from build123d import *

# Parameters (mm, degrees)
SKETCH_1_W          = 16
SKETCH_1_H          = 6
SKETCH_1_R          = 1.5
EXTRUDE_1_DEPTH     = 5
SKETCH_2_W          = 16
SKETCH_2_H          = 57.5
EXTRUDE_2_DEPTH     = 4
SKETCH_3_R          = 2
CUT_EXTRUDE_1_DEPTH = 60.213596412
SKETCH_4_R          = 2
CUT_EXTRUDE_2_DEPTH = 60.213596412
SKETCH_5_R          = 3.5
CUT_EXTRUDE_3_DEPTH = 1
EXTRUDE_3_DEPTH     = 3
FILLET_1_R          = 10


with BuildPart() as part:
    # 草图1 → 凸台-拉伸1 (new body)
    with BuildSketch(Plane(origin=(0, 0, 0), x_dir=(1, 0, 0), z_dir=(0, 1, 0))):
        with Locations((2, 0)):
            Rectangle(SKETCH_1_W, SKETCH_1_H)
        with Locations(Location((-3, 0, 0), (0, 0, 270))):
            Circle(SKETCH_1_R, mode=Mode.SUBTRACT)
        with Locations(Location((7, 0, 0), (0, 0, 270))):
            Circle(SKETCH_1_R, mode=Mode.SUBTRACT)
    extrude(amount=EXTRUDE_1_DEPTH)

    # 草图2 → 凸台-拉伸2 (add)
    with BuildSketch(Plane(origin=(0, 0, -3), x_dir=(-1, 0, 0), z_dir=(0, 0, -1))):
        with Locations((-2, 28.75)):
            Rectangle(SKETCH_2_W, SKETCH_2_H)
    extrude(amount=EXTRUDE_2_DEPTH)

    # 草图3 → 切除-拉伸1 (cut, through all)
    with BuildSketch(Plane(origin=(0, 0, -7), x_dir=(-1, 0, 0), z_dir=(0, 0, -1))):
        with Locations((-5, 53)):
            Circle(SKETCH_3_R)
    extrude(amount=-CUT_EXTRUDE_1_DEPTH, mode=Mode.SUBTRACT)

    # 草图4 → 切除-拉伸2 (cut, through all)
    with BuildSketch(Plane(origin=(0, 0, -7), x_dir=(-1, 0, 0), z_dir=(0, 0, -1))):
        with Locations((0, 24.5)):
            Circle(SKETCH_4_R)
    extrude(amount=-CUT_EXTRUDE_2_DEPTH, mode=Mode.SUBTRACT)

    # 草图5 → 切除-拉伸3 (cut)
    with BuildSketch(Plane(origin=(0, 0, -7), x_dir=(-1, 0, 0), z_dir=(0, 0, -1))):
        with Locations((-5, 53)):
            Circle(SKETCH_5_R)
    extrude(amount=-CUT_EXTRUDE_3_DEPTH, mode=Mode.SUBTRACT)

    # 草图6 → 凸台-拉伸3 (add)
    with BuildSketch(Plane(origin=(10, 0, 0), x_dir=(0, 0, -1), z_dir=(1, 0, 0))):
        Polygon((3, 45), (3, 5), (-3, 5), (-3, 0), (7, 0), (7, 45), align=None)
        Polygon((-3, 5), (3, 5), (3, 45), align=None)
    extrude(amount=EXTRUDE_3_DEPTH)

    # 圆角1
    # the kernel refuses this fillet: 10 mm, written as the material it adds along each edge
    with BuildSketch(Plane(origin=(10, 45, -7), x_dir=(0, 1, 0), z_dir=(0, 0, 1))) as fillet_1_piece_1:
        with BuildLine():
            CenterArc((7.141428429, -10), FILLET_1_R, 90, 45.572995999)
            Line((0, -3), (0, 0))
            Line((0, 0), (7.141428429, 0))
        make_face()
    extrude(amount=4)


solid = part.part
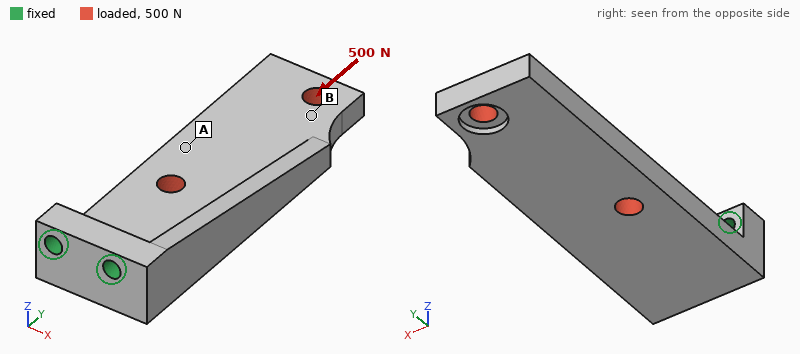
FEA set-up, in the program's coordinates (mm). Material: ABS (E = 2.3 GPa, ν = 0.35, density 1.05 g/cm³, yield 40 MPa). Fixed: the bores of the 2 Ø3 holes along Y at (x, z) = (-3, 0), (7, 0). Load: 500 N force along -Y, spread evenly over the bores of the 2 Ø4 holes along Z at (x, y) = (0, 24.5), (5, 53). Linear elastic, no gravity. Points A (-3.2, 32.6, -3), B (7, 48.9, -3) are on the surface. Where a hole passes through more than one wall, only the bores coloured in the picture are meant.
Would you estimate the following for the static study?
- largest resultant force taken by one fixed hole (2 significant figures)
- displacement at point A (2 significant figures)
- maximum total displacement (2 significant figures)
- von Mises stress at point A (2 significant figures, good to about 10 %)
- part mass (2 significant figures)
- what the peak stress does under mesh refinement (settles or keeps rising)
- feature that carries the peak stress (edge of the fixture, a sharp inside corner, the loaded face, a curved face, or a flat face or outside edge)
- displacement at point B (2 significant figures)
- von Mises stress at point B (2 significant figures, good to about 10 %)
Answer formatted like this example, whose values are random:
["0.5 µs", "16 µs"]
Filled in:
["250 N", "0.42 mm", "0.63 mm", "3.4 MPa", "5.2 g", "keeps rising", "edge of the fixture", "0.55 mm", "7.7 MPa"]
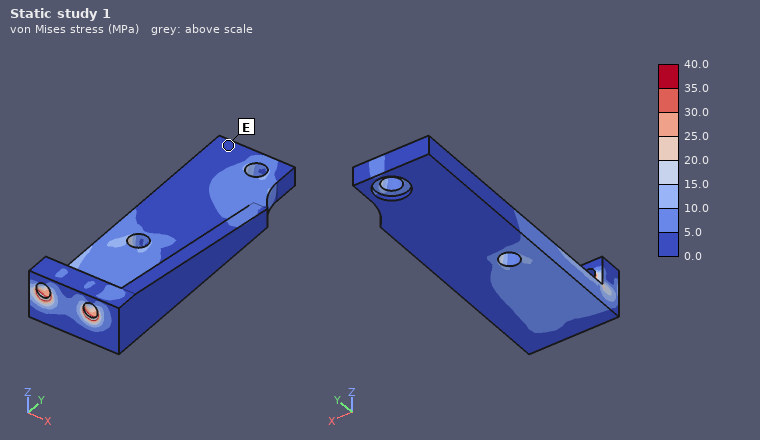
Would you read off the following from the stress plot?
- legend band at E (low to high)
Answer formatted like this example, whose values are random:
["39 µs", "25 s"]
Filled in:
["0.0 to 5.0 MPa"]
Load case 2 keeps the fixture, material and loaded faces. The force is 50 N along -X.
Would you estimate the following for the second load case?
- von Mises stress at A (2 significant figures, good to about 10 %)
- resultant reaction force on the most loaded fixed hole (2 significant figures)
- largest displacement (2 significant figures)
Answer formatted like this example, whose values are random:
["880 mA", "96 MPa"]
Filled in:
["1.8 MPa", "130 N", "0.65 mm"]
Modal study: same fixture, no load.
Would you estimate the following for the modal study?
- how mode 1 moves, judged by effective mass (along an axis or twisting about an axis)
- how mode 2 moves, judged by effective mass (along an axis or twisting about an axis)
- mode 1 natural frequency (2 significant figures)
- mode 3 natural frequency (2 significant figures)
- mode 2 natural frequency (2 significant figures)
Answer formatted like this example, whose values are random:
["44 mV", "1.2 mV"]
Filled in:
["along Z", "along X", "460 Hz", "2000 Hz", "1200 Hz"]
